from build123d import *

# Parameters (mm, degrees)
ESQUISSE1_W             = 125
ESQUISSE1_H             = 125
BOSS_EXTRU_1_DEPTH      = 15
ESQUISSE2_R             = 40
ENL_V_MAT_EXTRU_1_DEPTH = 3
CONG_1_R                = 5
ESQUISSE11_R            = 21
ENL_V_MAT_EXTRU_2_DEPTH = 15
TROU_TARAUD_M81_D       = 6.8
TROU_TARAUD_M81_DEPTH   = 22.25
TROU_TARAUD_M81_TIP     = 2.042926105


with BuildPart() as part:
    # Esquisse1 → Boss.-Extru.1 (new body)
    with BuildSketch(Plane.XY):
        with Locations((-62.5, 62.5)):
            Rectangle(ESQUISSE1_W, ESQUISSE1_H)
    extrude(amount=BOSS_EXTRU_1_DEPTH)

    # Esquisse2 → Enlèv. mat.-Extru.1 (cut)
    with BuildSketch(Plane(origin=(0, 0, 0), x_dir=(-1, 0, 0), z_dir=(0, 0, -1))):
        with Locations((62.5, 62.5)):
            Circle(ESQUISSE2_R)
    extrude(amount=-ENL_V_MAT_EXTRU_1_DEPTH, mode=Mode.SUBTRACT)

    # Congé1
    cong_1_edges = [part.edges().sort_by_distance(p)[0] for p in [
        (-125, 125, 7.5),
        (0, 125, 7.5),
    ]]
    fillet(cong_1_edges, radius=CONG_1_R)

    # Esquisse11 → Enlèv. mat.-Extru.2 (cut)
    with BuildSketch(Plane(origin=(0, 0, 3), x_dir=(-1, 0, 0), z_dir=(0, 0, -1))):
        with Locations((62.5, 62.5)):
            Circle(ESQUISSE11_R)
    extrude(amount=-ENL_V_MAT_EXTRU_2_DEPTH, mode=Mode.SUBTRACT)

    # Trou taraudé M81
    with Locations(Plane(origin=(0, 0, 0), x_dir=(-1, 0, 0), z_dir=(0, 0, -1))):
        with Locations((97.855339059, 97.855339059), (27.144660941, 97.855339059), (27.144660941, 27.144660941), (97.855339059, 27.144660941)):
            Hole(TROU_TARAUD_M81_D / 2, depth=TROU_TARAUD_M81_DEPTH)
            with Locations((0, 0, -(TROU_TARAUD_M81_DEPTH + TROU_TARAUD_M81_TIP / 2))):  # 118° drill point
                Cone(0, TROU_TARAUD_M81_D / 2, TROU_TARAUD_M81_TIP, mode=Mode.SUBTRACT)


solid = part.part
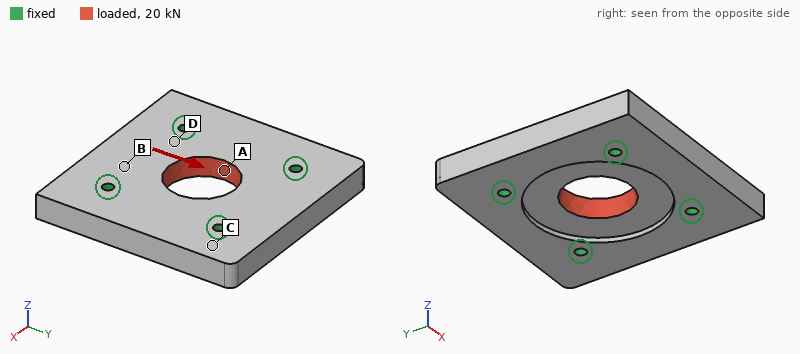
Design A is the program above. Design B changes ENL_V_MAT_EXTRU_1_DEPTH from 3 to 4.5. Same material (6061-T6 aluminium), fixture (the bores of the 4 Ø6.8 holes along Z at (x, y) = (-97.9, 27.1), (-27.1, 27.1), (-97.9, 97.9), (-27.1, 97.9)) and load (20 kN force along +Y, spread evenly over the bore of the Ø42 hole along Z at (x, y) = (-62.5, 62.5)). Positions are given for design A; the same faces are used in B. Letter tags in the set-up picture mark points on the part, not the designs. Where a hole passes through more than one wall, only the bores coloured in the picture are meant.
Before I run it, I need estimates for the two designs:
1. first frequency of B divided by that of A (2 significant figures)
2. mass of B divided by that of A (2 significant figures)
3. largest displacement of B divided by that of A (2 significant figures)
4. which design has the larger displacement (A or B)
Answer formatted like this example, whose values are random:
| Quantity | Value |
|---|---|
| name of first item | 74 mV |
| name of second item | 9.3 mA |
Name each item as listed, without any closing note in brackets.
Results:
| Quantity | Value |
|---|---|
| first frequency of B divided by that of A | 1.00 |
| mass of B divided by that of A | 0.97 |
| largest displacement of B divided by that of A | 1.1 |
| which design has the larger displacement | B |
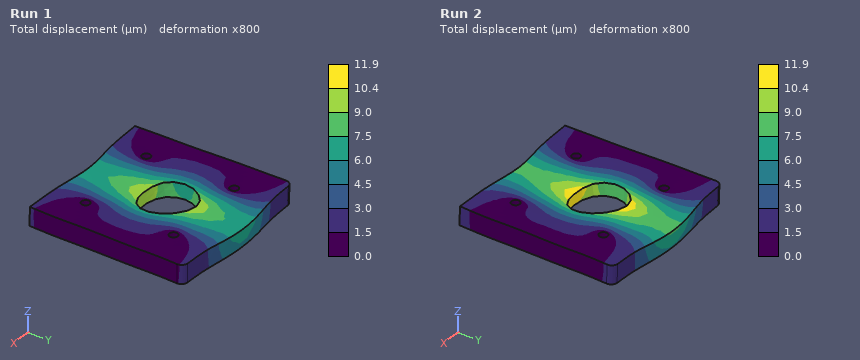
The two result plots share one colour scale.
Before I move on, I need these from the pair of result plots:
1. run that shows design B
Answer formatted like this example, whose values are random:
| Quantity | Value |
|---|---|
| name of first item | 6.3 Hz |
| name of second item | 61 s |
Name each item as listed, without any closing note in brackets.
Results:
| Quantity | Value |
|---|---|
| run that shows design B | Run 2 |
